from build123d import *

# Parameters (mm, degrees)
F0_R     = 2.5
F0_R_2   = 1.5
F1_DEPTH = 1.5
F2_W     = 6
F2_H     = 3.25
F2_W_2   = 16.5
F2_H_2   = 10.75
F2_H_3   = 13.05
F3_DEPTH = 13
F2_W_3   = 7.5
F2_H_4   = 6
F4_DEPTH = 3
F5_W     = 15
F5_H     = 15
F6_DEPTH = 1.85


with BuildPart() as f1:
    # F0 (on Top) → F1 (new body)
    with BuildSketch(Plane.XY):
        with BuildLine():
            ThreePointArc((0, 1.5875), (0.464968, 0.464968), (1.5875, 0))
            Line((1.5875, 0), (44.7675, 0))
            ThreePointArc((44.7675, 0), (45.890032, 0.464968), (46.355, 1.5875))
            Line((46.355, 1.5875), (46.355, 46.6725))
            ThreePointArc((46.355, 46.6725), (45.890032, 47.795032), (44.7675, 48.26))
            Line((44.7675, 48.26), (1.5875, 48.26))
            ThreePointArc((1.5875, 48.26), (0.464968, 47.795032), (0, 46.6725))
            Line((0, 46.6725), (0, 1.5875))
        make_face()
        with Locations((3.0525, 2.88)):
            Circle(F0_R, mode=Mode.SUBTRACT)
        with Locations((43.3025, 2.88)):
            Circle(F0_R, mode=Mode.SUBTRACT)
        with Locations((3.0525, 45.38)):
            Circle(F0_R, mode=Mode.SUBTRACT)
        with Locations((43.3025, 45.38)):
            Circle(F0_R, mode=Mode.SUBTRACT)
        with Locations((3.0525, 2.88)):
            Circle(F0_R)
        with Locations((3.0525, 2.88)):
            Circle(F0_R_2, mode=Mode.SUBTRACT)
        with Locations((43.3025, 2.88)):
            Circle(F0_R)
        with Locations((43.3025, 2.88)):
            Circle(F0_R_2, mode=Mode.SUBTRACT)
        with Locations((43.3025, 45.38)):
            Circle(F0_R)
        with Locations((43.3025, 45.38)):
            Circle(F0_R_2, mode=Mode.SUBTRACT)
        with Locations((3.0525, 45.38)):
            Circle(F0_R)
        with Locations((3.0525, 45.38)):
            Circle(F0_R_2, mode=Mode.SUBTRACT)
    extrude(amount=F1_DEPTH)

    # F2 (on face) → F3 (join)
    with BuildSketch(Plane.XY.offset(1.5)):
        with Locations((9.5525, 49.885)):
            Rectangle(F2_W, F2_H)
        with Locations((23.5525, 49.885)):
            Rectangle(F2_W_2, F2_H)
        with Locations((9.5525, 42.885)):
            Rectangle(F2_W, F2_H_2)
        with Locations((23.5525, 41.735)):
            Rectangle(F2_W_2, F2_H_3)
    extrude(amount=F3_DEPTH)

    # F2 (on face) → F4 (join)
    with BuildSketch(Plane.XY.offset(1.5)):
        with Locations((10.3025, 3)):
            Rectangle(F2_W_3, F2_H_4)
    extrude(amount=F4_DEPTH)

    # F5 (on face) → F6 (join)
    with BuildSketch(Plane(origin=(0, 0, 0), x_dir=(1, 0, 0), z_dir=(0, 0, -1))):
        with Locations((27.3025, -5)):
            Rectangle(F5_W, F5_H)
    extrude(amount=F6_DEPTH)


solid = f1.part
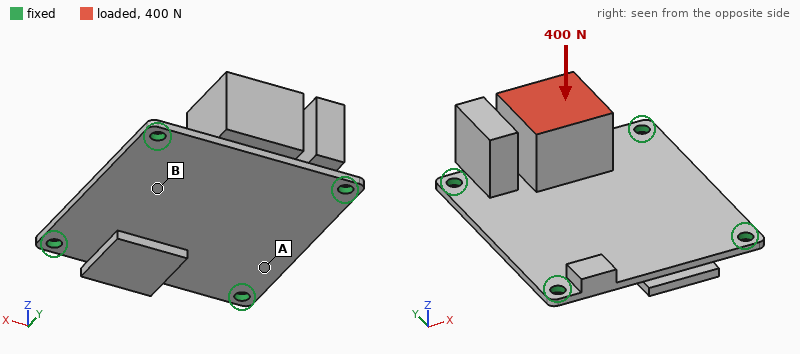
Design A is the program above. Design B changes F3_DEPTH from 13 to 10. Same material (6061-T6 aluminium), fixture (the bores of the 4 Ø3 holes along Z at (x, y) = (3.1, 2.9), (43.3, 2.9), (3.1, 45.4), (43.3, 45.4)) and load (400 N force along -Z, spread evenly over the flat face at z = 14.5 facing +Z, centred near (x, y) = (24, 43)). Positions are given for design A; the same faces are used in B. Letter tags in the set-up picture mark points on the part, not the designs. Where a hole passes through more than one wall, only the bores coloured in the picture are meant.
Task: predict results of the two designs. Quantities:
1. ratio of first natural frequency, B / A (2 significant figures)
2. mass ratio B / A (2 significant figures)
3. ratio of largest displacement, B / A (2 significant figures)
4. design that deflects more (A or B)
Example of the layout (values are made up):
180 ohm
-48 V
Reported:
1.1
0.87
0.84
A
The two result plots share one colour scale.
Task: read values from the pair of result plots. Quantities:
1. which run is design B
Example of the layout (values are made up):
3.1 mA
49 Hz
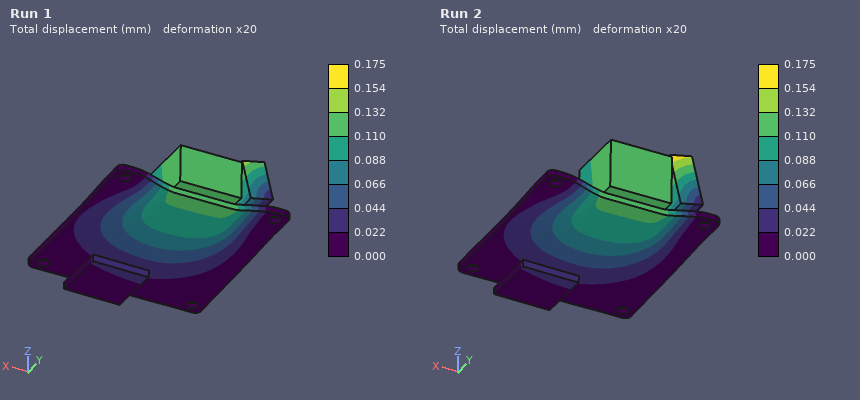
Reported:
Run 1
